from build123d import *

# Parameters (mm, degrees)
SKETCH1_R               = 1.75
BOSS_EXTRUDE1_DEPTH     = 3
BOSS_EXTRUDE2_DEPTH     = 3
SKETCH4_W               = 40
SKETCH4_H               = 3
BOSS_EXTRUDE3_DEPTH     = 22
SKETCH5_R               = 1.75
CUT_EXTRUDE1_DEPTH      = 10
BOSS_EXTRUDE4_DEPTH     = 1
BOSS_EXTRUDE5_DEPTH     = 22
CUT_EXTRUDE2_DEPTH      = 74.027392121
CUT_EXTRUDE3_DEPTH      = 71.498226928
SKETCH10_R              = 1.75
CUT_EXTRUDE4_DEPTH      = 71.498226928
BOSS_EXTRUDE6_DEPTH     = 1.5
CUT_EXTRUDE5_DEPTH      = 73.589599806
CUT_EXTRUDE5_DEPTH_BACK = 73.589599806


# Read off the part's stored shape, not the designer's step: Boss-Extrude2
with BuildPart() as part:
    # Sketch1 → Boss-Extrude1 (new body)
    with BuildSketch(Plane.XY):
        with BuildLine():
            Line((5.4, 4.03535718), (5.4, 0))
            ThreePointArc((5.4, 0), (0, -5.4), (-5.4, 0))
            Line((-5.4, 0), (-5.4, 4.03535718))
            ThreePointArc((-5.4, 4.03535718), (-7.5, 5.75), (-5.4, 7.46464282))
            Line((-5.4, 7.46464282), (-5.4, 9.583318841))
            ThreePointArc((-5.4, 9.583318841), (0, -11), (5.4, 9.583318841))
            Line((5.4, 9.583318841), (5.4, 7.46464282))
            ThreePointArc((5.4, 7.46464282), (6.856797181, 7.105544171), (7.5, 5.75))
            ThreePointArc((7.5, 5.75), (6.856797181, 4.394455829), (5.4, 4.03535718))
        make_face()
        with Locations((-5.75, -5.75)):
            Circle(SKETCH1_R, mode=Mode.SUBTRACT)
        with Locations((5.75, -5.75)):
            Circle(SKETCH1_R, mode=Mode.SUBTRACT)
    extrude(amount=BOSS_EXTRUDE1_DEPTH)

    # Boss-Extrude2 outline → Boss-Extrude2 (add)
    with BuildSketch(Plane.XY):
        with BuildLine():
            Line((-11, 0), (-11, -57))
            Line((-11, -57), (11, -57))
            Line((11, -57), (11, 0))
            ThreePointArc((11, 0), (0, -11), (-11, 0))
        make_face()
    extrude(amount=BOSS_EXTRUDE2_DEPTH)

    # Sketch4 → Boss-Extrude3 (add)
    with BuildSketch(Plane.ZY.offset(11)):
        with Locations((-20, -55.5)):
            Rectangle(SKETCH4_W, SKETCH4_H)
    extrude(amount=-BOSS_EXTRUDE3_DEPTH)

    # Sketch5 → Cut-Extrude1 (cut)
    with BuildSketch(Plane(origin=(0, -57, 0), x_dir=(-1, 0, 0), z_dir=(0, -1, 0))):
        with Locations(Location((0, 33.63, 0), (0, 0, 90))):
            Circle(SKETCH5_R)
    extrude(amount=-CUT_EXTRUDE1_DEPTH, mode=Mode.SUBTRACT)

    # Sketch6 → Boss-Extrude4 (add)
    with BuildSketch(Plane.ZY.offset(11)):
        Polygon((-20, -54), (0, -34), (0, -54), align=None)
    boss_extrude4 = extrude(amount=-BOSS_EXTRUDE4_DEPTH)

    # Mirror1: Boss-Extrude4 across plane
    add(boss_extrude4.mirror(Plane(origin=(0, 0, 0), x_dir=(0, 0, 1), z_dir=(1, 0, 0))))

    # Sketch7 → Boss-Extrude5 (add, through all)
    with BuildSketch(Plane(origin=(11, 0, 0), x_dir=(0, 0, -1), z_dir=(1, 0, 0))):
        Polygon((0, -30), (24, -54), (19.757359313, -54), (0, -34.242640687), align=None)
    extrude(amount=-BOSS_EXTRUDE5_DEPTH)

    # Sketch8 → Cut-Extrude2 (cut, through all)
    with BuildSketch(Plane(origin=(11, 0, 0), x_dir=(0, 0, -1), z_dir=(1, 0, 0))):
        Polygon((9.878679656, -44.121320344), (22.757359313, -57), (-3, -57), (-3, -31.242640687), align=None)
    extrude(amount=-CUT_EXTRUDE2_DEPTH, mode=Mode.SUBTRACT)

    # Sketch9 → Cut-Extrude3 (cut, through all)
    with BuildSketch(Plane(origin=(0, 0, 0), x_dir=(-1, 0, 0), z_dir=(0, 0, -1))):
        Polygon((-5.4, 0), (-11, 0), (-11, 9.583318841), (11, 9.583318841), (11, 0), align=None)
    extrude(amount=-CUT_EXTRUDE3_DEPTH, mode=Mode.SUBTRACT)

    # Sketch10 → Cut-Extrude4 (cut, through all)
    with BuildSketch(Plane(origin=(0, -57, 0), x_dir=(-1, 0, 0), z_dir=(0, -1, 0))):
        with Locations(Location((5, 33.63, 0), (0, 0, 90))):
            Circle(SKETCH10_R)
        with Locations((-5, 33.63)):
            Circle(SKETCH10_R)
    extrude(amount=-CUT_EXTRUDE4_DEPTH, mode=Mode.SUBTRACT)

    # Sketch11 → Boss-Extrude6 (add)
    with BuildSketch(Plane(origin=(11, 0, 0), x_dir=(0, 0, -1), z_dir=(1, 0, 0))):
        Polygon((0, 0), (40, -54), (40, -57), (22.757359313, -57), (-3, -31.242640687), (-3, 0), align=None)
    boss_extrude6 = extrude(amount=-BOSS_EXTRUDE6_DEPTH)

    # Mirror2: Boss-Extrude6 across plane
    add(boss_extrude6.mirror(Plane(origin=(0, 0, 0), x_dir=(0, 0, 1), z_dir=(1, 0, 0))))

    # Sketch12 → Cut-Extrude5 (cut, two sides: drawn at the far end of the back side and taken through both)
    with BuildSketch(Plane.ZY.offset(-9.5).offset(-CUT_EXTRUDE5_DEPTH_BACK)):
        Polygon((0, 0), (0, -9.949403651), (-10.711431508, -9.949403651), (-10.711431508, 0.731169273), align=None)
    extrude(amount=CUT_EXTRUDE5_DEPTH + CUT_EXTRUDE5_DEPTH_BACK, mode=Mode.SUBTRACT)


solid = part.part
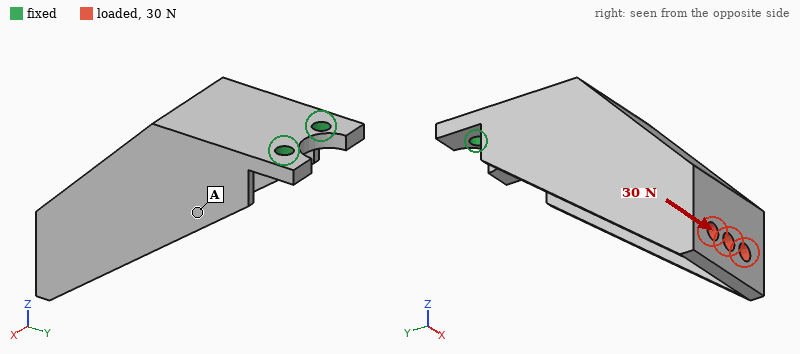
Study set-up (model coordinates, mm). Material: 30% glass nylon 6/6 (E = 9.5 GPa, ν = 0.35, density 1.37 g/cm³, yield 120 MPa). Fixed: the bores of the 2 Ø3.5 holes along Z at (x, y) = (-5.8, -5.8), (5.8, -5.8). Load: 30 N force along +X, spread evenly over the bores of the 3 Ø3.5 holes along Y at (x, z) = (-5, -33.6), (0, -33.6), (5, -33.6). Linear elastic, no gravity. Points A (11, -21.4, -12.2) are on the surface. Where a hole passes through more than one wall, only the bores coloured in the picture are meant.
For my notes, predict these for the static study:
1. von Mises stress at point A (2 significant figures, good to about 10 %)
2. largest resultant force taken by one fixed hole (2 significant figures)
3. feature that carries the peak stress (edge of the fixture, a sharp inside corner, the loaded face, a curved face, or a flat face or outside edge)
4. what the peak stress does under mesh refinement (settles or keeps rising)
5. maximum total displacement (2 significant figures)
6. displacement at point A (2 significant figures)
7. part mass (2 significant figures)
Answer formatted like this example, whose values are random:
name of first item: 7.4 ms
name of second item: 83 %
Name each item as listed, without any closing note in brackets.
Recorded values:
von Mises stress at point A: 6.6 MPa
largest resultant force taken by one fixed hole: 120 N
feature that carries the peak stress: edge of the fixture
what the peak stress does under mesh refinement: keeps rising
maximum total displacement: 0.89 mm
displacement at point A: 0.22 mm
part mass: 10 g
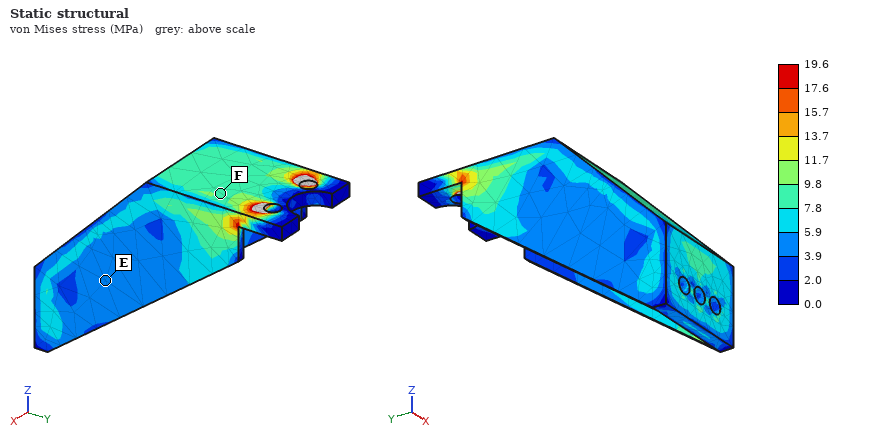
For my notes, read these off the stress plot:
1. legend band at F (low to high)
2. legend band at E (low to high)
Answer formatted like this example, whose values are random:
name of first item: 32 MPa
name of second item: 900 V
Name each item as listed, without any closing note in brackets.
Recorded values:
legend band at F: 7.8 to 9.8 MPa
legend band at E: 3.9 to 5.9 MPa
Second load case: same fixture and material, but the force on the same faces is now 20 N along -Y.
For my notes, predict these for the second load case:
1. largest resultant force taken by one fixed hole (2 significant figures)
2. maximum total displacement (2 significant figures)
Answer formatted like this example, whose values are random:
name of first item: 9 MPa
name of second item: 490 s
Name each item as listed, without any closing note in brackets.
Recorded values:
largest resultant force taken by one fixed hole: 15 N
maximum total displacement: 0.73 mm
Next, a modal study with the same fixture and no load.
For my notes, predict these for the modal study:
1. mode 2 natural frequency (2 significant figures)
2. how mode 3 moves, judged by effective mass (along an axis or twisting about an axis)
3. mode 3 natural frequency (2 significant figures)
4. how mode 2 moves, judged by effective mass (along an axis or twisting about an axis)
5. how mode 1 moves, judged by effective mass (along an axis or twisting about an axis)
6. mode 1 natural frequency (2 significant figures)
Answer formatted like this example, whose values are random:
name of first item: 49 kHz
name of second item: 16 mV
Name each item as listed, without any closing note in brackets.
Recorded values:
mode 2 natural frequency: 610 Hz
how mode 3 moves, judged by effective mass: along X
mode 3 natural frequency: 2700 Hz
how mode 2 moves, judged by effective mass: along X
how mode 1 moves, judged by effective mass: along Z
mode 1 natural frequency: 360 Hz
